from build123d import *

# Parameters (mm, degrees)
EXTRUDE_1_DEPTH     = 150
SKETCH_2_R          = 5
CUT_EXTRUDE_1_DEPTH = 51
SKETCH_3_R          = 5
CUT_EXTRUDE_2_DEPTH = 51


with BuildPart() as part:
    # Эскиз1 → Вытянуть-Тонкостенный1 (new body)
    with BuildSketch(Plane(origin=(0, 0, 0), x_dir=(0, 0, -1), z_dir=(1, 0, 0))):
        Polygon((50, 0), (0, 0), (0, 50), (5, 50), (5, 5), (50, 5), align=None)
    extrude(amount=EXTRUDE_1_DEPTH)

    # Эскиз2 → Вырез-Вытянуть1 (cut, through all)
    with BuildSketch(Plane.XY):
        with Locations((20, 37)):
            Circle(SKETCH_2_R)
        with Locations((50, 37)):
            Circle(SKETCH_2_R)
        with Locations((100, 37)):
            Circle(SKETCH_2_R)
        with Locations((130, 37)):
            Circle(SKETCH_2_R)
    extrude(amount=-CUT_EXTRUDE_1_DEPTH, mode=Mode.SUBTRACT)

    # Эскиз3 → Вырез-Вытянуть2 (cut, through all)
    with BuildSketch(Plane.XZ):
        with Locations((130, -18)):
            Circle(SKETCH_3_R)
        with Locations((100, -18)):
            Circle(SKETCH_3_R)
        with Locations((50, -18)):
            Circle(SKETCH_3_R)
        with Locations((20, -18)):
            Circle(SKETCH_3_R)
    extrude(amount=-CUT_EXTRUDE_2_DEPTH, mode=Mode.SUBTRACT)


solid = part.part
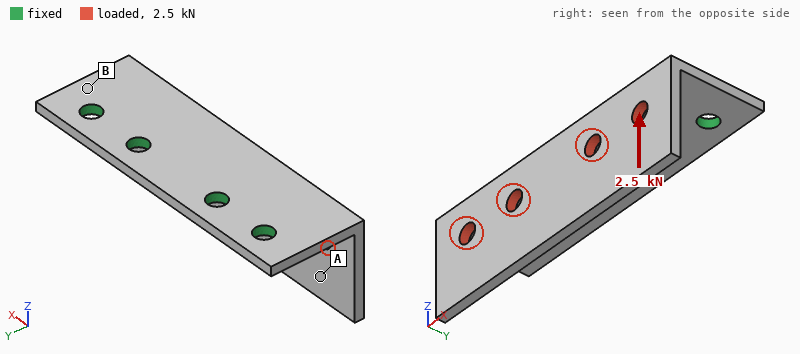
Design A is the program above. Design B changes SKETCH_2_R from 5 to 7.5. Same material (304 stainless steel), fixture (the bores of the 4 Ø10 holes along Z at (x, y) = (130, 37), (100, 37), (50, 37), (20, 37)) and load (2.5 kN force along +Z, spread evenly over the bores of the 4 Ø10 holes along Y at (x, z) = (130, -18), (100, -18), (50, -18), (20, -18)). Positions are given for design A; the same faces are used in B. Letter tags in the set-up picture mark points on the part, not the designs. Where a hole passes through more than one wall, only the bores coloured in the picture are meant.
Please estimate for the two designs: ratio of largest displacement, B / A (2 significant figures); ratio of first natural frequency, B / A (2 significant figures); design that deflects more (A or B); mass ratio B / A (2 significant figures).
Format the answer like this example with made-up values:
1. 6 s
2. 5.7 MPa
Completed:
1. 0.80
2. 1.1
3. A
4. 0.97
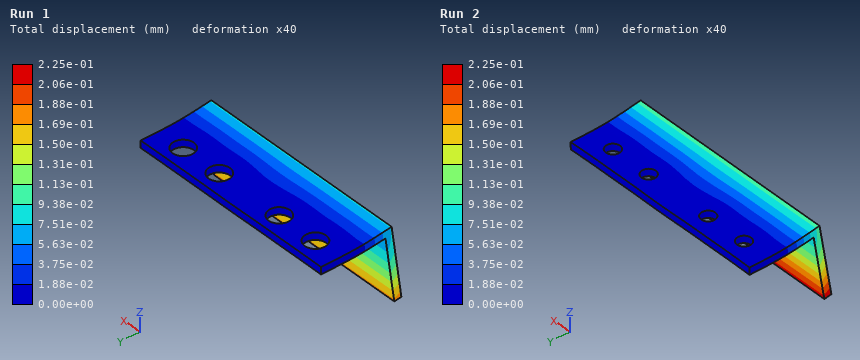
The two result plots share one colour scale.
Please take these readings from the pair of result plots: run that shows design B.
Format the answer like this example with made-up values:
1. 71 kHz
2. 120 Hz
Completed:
1. Run 1
